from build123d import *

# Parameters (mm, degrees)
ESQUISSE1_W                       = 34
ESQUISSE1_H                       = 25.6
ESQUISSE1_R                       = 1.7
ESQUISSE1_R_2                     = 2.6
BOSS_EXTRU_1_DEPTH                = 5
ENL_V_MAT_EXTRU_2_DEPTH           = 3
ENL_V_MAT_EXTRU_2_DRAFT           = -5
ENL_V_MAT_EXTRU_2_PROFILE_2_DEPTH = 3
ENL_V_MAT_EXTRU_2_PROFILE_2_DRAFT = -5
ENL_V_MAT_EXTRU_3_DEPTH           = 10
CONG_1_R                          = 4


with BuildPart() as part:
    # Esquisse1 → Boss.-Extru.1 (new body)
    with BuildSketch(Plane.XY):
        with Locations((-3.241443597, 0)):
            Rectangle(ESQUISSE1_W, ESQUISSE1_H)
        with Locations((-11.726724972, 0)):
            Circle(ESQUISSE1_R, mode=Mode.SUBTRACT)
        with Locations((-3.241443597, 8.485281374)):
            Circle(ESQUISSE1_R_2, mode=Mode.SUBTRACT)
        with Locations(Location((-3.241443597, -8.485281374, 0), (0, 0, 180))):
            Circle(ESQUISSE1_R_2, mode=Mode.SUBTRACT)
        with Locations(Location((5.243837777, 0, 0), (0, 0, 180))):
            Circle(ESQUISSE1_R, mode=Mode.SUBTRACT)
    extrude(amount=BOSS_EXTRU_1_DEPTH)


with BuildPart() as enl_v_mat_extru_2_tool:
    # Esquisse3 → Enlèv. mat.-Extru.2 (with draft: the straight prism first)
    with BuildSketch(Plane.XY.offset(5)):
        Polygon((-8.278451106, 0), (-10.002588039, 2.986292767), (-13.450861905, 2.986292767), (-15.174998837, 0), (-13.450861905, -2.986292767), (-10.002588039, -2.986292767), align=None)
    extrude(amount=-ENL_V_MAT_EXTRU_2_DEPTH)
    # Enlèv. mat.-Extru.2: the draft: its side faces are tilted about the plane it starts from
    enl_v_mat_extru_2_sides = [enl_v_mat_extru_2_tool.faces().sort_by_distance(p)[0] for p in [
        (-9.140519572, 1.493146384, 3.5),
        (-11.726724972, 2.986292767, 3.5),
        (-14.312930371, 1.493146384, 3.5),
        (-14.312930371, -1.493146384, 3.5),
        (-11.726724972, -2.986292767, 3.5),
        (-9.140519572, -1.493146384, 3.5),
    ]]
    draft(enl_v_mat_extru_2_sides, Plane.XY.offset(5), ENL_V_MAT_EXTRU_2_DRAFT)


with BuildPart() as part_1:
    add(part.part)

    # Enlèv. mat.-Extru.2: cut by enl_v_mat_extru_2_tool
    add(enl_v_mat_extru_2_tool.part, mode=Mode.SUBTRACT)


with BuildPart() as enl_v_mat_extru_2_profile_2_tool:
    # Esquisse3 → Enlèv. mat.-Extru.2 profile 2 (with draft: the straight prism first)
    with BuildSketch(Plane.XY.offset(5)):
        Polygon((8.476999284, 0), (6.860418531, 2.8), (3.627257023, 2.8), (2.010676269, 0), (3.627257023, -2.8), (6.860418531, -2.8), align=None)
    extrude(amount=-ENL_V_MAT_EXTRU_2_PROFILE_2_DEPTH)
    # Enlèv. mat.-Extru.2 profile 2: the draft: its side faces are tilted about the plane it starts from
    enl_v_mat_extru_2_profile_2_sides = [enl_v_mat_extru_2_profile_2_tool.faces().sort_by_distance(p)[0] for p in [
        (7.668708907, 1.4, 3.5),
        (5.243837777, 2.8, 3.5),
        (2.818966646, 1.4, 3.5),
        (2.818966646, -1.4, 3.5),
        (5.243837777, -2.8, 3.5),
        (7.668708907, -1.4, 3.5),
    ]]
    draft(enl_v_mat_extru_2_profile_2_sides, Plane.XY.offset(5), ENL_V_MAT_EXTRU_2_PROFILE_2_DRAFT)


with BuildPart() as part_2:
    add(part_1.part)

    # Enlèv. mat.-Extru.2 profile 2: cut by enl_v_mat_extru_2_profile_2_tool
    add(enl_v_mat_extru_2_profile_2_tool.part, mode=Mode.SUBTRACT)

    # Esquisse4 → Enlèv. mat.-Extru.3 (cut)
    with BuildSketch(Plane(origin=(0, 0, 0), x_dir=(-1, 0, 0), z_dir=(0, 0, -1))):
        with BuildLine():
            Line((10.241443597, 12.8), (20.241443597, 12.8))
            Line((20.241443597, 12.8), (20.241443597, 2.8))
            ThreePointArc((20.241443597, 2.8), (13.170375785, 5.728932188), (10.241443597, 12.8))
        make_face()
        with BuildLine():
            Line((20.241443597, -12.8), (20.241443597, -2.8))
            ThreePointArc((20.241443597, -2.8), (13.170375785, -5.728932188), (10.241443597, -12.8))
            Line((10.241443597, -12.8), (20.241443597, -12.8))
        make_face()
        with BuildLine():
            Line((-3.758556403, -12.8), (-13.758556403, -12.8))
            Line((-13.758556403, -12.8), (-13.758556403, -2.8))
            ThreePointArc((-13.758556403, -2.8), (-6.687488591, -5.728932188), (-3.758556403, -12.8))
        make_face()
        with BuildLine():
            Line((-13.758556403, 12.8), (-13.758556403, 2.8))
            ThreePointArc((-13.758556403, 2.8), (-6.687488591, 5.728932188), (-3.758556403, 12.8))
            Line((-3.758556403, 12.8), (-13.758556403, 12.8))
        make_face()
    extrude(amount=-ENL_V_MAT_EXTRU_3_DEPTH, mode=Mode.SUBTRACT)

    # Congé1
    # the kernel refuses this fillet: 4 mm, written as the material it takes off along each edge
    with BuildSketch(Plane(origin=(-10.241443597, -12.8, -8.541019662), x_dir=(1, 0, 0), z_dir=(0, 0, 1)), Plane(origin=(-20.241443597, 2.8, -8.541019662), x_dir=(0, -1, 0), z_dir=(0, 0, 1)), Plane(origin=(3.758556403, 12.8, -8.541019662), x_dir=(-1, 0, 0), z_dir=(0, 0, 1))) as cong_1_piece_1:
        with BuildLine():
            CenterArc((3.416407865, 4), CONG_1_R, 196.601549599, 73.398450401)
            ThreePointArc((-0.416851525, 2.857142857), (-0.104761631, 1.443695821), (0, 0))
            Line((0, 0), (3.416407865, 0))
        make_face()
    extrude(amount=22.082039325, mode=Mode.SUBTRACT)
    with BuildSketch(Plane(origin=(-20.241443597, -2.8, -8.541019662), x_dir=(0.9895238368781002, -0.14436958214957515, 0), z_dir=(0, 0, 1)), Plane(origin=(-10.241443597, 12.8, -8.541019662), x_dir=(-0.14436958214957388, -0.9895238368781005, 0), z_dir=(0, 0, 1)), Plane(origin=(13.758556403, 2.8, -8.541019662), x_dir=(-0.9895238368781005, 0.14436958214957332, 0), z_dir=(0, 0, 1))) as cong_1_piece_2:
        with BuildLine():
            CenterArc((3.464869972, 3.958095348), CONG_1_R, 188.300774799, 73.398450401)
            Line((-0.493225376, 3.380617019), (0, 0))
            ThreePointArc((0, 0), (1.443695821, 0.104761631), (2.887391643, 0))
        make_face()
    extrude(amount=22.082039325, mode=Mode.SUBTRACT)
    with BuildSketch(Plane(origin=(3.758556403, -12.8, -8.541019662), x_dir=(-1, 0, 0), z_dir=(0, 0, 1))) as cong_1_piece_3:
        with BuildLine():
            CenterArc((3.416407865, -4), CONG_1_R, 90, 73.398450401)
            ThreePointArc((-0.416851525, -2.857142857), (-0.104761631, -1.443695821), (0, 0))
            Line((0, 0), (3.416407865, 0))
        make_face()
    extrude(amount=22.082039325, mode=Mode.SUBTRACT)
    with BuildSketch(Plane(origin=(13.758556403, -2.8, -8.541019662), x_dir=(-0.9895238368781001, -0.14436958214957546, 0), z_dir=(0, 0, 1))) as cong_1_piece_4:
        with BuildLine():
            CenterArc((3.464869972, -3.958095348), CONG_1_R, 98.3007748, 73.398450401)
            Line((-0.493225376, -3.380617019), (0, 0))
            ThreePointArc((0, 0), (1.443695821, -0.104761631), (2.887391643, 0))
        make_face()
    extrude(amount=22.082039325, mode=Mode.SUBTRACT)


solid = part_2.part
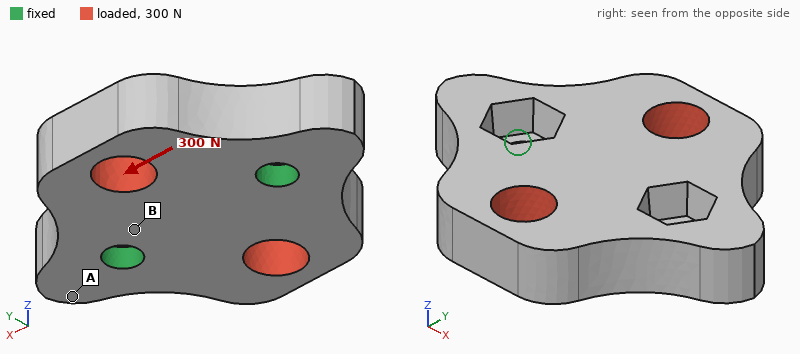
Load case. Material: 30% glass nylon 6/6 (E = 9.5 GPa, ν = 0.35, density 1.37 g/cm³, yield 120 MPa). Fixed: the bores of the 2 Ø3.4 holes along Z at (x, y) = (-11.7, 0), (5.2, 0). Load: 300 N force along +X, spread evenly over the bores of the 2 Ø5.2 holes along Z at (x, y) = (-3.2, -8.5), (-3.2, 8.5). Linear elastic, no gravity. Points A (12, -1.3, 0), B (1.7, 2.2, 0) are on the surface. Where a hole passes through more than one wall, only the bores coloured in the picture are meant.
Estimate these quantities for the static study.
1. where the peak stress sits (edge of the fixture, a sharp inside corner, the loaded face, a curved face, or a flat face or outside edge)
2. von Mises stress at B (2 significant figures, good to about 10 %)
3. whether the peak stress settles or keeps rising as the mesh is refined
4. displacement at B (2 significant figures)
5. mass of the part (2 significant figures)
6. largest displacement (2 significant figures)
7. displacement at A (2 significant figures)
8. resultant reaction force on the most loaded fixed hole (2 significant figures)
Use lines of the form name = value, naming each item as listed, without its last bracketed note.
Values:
where the peak stress sits = edge of the fixture
von Mises stress at B = 4.5 MPa
whether the peak stress settles or keeps rising as the mesh is refined = keeps rising
displacement at B = 1.8 µm
mass of the part = 3.1 g
largest displacement = 9.6 µm
displacement at A = 4.0 µm
resultant reaction force on the most loaded fixed hole = 150 N
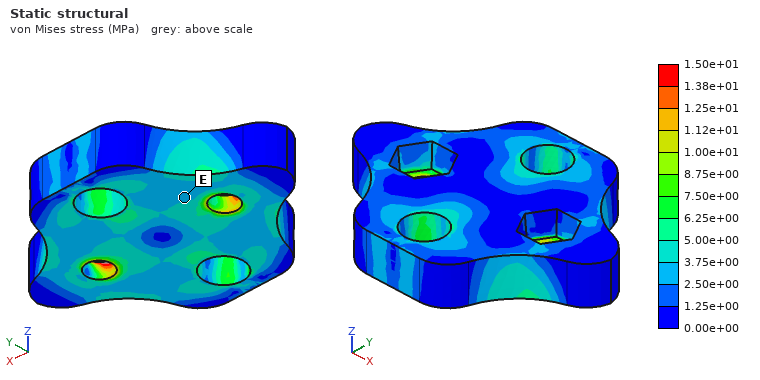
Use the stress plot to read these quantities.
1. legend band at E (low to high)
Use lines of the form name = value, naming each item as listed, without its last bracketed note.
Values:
legend band at E = 2.50e+00 to 3.75e+00 MPa
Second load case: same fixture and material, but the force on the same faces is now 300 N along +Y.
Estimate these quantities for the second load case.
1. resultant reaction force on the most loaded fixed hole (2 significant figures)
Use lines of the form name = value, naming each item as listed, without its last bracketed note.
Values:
resultant reaction force on the most loaded fixed hole = 150 N
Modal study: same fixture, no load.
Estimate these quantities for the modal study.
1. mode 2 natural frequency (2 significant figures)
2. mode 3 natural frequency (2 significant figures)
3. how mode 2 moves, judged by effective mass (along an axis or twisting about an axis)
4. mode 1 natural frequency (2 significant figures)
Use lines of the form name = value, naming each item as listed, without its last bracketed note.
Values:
mode 2 natural frequency = 12 kHz
mode 3 natural frequency = 19 kHz
how mode 2 moves, judged by effective mass = along Z
mode 1 natural frequency = 6600 Hz
